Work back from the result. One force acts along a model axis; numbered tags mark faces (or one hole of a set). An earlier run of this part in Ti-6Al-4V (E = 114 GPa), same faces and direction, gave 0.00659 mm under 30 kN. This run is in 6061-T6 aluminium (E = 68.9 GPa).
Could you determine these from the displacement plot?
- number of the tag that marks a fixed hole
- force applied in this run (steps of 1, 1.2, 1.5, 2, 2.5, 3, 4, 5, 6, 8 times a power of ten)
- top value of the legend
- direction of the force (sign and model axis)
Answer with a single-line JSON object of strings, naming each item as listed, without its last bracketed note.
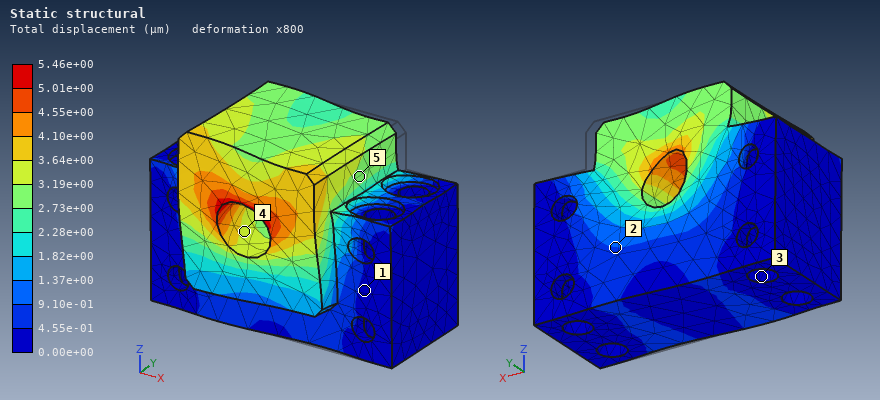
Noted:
{"number of the tag that marks a fixed hole": "3", "force applied in this run": "15 kN", "top value of the legend": "5.46e+00 µm", "direction of the force": "-X"}
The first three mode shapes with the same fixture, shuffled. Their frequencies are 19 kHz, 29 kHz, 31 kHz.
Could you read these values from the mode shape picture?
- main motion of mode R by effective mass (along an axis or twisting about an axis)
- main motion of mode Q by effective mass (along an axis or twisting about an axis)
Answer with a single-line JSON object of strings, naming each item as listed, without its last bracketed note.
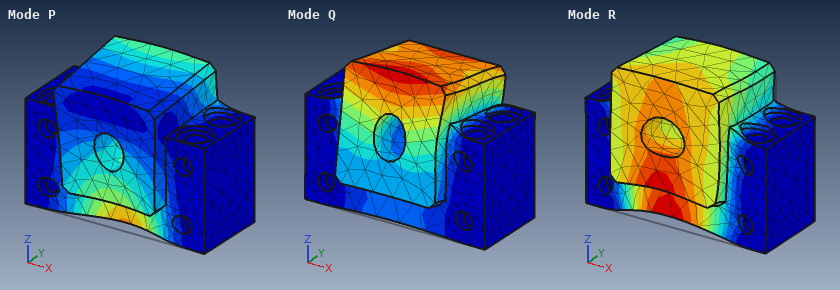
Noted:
{"main motion of mode R by effective mass": "along Z", "main motion of mode Q by effective mass": "along Y"}
